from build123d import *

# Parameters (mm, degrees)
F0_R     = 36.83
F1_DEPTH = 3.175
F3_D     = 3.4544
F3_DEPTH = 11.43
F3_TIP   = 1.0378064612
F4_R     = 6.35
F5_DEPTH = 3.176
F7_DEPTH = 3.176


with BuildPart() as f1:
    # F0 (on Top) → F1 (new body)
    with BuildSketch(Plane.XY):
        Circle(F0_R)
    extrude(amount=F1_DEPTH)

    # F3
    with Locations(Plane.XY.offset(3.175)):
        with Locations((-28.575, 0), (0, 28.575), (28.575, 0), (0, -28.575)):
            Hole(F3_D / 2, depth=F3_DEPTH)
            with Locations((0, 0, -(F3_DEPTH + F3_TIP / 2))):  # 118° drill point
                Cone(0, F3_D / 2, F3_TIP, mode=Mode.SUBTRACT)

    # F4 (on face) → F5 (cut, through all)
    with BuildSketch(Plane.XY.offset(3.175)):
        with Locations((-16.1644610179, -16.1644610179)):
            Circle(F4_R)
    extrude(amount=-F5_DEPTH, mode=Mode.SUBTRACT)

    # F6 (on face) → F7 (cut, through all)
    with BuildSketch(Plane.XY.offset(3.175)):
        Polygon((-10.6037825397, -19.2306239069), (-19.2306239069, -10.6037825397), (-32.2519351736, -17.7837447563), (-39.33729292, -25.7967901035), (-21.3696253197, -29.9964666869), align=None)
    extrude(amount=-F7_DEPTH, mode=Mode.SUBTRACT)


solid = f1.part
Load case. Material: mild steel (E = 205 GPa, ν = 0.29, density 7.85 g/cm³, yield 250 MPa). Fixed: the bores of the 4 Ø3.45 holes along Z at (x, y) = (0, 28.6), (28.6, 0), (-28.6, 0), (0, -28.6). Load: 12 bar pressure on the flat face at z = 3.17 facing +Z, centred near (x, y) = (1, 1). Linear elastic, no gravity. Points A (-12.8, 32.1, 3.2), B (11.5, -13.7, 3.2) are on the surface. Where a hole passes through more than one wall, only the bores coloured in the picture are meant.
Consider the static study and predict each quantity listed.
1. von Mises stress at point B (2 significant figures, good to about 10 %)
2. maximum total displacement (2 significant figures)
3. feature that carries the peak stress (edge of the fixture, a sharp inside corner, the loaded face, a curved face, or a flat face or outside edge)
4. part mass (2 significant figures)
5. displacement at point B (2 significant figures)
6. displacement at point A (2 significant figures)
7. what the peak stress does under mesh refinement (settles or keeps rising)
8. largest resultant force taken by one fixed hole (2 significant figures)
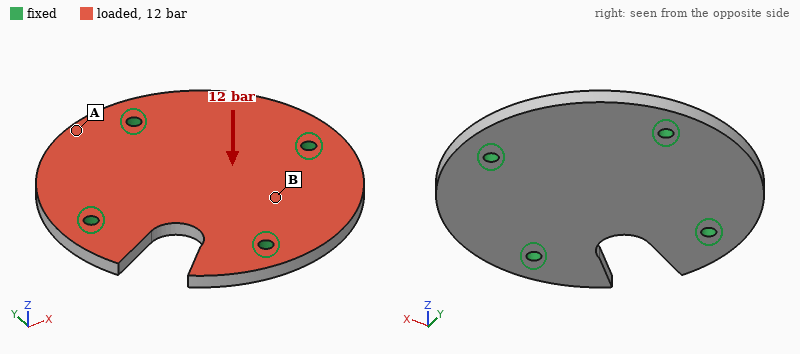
63 MPa
32 µm
edge of the fixture
99 g
23 µm
14 µm
keeps rising
1.3 kN
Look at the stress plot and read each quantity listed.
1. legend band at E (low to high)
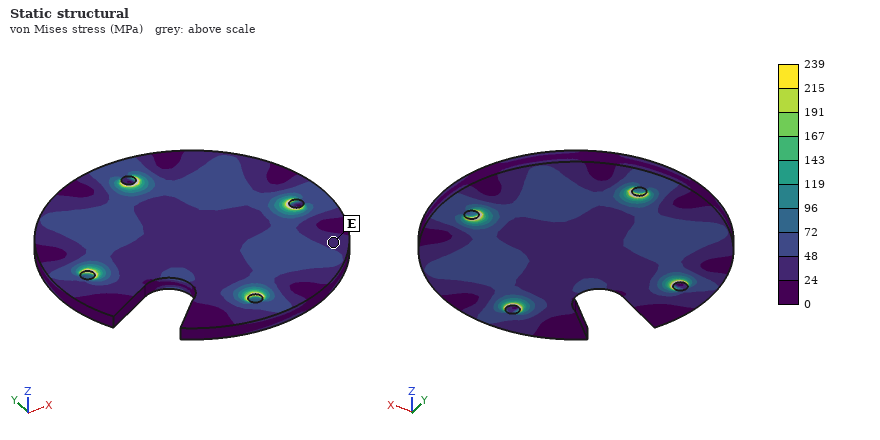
24 to 48 MPa
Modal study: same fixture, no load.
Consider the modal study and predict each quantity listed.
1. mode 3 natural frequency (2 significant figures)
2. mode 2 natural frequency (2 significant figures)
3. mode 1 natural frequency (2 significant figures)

7200 Hz
7200 Hz
6900 Hz
